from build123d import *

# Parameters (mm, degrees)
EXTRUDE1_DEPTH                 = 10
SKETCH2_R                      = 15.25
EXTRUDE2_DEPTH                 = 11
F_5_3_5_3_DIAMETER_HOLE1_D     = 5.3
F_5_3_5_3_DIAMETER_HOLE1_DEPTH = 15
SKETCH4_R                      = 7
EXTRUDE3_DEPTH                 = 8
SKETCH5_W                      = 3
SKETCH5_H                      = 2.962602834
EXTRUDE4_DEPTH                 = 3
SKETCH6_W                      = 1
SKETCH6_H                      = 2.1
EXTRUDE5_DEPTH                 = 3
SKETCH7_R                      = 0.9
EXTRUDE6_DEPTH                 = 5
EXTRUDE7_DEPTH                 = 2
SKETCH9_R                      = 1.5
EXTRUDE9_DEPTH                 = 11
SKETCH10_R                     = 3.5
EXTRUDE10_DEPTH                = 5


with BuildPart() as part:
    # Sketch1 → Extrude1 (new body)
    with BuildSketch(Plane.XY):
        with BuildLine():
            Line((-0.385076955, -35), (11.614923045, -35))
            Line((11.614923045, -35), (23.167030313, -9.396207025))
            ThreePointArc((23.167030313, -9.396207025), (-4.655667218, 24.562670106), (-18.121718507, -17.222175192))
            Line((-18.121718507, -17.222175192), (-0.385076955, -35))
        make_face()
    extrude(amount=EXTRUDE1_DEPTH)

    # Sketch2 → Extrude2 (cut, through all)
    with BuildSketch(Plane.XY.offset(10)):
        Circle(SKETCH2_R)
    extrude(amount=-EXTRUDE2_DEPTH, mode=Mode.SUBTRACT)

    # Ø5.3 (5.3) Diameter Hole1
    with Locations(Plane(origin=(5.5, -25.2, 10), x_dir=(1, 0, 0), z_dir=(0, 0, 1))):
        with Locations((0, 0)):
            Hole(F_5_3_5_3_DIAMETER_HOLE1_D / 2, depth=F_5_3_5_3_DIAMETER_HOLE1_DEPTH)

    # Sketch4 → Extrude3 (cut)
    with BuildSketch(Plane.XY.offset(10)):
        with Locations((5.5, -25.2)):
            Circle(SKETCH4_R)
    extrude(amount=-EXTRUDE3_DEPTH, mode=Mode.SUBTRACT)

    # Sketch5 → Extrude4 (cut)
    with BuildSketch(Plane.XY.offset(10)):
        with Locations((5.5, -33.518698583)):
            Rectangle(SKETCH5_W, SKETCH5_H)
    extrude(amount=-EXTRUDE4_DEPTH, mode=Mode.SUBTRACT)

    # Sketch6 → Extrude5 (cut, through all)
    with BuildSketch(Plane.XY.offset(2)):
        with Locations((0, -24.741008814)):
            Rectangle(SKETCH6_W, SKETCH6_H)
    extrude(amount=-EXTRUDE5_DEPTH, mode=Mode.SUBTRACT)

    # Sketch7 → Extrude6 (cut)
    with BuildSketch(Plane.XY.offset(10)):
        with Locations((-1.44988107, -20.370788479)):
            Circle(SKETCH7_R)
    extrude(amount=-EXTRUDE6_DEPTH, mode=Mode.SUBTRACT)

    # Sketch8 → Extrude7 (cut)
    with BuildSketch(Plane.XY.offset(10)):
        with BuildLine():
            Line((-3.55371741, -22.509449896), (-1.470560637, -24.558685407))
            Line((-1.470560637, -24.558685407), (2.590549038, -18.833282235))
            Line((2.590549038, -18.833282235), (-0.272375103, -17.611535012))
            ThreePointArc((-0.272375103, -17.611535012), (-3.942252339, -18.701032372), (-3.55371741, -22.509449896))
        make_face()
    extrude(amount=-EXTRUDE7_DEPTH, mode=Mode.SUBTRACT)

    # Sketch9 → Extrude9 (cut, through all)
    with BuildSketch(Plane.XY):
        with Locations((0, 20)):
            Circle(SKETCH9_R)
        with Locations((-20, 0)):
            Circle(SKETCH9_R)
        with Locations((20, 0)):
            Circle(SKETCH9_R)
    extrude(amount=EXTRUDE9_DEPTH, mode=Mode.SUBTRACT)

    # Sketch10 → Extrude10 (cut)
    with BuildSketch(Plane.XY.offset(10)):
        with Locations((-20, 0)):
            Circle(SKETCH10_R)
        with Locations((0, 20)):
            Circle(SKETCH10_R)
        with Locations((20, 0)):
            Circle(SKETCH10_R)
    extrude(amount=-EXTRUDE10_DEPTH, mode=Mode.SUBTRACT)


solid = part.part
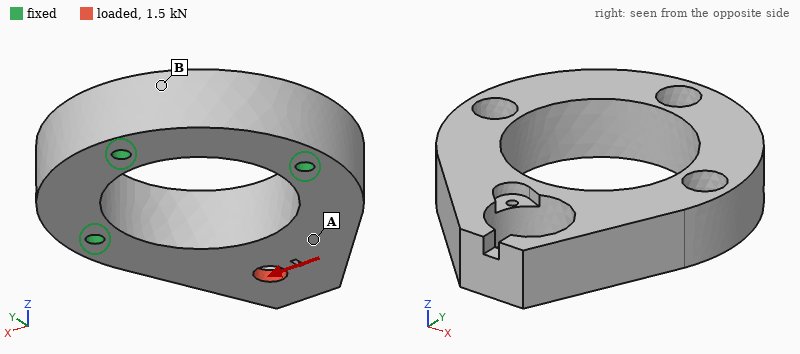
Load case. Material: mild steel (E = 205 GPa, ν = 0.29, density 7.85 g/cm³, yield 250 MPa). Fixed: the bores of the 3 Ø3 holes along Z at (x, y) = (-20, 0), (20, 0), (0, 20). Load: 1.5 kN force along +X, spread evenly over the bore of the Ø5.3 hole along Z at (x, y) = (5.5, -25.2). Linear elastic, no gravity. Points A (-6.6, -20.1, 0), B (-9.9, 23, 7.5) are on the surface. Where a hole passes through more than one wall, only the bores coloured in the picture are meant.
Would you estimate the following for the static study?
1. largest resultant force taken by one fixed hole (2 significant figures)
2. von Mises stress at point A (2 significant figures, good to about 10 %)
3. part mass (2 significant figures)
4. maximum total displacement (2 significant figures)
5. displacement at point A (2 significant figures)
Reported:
1.1 kN
23 MPa
100 g
9.4 µm
6.0 µm
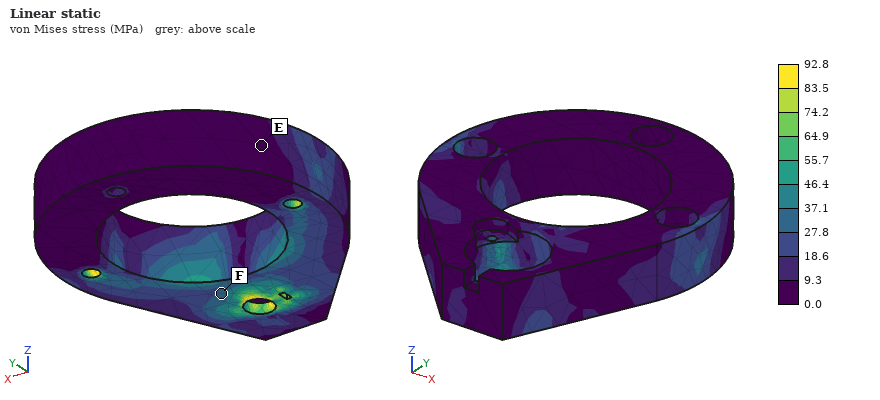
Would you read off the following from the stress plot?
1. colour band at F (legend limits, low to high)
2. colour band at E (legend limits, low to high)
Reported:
27.8 to 37.1 MPa
0.0 to 9.3 MPa
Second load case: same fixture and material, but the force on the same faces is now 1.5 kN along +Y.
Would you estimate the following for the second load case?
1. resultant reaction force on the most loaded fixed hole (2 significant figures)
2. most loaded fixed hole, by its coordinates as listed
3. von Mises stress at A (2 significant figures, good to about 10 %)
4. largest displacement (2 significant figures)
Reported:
1.0 kN
(20, 0)
21 MPa
16 µm
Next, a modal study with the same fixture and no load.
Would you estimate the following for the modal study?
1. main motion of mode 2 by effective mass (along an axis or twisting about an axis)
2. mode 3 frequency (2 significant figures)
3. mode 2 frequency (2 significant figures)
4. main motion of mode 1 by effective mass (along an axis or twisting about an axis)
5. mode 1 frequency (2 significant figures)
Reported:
along X
13 kHz
13 kHz
along Z
4500 Hz
